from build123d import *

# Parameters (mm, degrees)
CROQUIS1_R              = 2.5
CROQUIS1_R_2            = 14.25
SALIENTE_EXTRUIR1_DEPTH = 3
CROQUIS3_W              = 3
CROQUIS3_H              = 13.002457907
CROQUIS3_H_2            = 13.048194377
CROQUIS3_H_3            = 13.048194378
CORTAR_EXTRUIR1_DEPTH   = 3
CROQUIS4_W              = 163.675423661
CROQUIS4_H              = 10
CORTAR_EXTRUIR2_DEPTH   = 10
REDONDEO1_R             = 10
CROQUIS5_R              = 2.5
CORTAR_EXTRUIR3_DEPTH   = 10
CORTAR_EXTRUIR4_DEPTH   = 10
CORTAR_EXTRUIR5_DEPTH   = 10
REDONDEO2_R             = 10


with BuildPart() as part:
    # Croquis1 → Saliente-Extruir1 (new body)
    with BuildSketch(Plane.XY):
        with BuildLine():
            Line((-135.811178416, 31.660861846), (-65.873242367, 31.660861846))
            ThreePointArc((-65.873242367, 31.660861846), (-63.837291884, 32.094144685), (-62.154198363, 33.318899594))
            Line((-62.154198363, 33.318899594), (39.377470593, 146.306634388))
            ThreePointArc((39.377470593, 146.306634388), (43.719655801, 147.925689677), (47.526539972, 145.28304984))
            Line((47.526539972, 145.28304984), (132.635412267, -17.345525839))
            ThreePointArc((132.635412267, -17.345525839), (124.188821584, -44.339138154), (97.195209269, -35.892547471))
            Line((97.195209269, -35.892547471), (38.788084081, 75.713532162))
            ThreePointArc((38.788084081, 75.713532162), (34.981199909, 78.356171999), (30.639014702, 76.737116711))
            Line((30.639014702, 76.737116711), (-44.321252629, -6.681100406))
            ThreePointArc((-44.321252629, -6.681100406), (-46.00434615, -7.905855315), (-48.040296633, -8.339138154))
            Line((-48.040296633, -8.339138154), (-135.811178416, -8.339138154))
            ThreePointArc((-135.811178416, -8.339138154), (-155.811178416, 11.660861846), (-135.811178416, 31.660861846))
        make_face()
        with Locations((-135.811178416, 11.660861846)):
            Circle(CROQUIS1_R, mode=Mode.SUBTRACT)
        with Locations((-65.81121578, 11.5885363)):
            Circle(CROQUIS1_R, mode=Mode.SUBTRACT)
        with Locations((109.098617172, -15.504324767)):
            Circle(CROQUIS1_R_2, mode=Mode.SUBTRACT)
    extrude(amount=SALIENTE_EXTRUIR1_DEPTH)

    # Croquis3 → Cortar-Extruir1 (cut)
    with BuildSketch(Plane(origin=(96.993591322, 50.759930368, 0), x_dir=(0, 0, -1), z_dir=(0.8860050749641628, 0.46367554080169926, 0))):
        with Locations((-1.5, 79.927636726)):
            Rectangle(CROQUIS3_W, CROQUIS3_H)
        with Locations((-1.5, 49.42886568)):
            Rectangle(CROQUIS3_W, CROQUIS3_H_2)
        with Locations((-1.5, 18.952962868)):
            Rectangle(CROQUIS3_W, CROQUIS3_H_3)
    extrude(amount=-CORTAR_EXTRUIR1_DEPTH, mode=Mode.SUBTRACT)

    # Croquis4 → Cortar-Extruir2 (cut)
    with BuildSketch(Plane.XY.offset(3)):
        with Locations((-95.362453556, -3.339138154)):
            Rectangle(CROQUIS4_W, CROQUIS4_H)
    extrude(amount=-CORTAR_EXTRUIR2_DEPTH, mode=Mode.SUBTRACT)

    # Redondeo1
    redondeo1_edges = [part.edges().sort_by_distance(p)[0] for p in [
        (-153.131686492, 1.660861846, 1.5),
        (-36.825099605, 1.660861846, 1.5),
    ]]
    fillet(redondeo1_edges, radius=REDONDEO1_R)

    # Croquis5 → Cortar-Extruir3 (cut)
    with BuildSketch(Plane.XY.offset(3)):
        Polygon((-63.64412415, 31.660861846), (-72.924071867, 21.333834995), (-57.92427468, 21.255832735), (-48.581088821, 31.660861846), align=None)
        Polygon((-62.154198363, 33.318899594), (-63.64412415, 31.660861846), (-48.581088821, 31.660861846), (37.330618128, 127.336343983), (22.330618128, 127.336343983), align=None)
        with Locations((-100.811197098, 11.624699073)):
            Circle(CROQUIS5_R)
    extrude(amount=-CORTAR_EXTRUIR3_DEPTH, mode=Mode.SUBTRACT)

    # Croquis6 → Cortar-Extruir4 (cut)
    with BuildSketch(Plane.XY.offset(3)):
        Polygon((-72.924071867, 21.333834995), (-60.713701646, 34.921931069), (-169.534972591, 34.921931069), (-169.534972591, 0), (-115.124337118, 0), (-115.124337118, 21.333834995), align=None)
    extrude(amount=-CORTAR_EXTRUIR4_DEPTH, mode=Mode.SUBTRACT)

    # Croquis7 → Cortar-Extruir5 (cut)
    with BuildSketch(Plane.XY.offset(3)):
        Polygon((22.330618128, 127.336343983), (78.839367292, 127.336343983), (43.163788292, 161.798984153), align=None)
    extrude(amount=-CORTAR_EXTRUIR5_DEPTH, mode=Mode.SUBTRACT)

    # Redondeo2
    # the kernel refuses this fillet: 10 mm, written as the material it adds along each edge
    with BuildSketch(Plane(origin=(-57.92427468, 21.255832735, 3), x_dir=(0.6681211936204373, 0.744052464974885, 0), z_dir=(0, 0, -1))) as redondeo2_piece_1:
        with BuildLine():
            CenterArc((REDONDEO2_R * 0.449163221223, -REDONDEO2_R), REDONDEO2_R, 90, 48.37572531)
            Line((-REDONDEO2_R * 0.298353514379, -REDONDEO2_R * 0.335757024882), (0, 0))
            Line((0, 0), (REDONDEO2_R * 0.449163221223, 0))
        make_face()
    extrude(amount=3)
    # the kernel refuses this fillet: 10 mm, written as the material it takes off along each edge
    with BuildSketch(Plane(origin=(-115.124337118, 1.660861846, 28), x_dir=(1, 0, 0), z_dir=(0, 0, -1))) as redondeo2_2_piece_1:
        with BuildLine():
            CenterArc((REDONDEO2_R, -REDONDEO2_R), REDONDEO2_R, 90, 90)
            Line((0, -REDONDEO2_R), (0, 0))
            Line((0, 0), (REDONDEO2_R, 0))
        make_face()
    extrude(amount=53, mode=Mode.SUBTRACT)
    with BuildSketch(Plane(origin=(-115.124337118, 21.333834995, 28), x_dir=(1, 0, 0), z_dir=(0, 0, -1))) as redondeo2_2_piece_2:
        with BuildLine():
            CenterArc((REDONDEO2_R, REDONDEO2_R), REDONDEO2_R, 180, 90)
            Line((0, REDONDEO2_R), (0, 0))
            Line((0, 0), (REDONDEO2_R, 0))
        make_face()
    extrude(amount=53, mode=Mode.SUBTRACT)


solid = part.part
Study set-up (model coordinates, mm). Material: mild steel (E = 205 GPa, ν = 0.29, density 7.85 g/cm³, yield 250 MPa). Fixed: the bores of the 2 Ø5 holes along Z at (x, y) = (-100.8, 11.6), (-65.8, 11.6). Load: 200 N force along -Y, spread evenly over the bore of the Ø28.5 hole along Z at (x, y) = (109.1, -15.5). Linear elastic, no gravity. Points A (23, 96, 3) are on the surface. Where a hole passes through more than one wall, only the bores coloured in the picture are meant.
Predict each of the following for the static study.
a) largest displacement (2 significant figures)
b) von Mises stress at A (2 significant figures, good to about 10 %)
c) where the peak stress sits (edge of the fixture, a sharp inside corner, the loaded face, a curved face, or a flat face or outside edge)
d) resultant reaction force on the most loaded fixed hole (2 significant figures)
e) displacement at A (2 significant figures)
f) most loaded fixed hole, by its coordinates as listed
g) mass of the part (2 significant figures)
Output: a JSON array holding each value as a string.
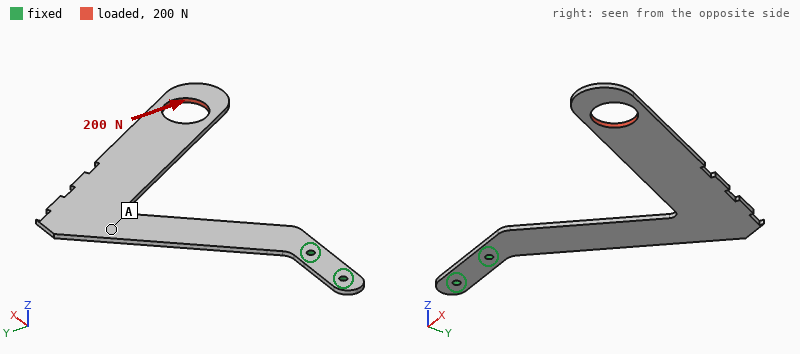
["0.81 mm", "16 MPa", "edge of the fixture", "820 N", "0.37 mm", "(-65.8, 11.6)", "260 g"]
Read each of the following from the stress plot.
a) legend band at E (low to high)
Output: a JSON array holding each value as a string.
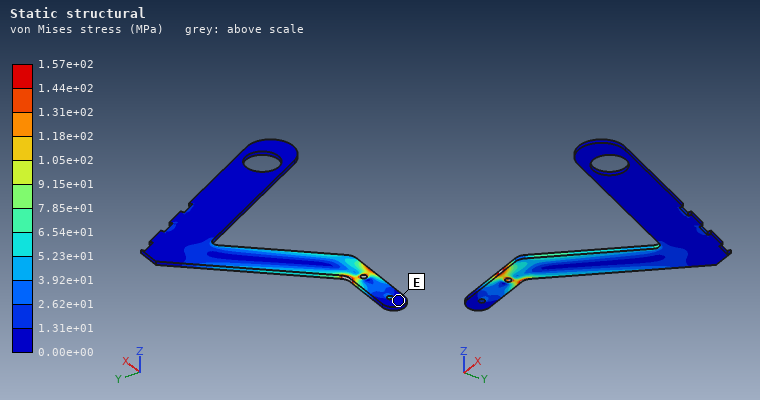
["0.00e+00 to 1.31e+01 MPa"]
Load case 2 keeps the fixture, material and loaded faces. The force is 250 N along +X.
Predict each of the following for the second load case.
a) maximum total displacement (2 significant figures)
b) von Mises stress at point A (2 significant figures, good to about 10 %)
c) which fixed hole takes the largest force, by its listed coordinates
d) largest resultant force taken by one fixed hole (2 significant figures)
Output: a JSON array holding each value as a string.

["0.44 mm", "23 MPa", "(-65.8, 11.6)", "260 N"]
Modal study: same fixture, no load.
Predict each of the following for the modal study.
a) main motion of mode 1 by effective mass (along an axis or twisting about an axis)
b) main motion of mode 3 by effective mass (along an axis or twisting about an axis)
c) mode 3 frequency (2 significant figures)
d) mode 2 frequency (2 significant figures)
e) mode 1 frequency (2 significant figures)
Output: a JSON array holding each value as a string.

["along Z", "along Y", "250 Hz", "83 Hz", "39 Hz"]
